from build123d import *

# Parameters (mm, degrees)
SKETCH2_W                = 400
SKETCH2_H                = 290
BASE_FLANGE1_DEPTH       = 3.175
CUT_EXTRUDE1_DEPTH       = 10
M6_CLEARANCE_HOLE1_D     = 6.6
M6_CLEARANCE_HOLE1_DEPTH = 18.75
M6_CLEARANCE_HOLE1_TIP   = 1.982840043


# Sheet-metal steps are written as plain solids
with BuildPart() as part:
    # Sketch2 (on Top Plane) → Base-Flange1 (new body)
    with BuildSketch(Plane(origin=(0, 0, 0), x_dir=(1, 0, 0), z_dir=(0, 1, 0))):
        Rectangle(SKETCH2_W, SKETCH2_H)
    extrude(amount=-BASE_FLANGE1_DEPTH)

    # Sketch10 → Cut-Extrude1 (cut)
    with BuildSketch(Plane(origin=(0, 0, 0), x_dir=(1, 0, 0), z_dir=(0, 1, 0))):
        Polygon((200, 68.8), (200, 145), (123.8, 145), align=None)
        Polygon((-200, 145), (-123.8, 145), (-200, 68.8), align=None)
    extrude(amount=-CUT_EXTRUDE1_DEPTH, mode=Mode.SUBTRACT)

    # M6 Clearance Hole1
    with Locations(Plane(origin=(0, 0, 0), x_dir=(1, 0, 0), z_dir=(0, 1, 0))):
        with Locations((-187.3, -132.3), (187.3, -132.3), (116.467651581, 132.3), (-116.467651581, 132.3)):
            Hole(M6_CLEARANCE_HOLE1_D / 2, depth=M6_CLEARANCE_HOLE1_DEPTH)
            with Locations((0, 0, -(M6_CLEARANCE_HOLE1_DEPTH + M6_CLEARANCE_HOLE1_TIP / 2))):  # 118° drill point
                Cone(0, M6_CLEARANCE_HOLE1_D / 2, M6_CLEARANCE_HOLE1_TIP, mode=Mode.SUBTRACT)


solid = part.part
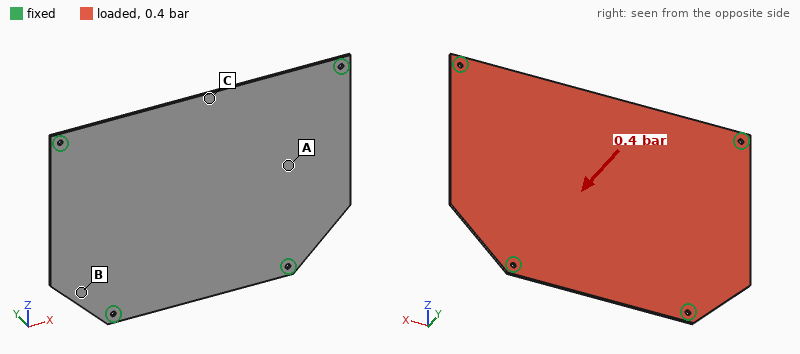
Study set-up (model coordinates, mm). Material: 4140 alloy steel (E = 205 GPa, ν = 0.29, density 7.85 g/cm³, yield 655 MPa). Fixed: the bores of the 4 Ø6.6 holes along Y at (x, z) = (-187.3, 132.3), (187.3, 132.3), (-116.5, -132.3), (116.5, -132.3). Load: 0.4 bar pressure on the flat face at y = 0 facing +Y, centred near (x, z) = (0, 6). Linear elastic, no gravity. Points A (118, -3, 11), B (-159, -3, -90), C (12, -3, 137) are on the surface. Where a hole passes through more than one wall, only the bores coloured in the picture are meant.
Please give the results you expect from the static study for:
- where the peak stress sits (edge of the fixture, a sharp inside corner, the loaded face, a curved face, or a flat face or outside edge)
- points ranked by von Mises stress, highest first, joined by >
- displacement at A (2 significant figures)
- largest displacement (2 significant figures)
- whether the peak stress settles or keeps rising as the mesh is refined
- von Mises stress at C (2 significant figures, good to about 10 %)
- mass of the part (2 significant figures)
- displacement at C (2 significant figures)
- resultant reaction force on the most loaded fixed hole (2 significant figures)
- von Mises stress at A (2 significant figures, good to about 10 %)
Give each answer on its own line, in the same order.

edge of the fixture
C > A > B
2.9 mm
5.4 mm
keeps rising
170 MPa
2.7 kg
5.3 mm
1.1 kN
110 MPa
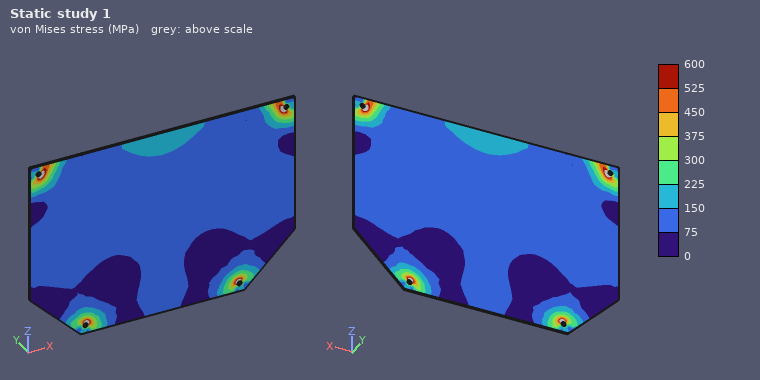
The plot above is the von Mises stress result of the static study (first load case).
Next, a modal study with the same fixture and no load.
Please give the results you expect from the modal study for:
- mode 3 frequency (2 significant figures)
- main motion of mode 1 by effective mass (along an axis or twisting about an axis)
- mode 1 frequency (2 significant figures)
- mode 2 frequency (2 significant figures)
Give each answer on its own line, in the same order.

200 Hz
along Y
110 Hz
200 Hz
